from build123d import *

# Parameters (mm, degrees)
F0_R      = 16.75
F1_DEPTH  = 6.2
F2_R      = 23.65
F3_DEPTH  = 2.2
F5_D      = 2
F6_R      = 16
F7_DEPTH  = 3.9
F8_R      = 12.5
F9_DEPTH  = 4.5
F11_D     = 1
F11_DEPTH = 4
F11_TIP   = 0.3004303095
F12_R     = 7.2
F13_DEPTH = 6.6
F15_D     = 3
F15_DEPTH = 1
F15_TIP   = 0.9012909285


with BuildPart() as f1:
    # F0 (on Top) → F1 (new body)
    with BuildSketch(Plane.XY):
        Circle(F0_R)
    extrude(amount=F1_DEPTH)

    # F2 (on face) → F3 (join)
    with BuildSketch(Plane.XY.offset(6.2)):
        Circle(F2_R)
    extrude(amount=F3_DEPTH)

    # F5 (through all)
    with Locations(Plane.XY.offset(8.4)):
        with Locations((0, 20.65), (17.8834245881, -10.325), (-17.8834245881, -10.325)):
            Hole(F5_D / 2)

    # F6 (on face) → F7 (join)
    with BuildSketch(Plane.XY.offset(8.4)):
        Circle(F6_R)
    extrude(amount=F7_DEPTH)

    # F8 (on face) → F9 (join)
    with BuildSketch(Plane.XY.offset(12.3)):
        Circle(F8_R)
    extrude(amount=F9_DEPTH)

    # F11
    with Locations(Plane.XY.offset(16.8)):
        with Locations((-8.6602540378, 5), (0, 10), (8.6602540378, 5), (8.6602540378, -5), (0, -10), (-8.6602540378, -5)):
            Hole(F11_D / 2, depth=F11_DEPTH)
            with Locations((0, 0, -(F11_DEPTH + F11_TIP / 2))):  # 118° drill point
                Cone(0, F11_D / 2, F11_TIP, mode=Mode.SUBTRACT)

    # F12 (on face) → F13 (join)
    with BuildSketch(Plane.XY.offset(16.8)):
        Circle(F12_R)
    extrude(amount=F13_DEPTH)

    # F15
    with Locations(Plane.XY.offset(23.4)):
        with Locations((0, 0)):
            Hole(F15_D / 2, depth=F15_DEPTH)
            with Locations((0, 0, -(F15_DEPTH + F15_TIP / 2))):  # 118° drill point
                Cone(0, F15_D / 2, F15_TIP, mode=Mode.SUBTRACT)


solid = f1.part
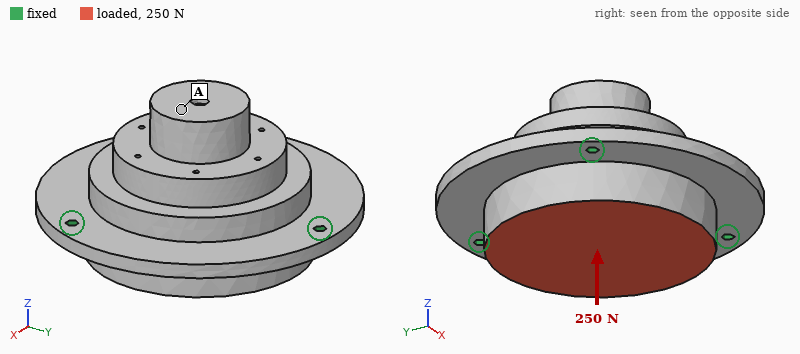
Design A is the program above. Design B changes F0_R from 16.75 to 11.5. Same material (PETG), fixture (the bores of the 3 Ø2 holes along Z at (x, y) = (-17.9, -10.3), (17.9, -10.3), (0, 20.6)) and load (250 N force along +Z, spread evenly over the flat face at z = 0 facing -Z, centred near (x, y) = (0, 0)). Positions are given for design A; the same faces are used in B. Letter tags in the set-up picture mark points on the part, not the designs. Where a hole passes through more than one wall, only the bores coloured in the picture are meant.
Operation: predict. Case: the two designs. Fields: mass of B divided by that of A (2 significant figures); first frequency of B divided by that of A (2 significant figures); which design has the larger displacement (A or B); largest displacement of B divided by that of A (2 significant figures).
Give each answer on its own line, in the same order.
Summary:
0.82
0.90
B
1.6
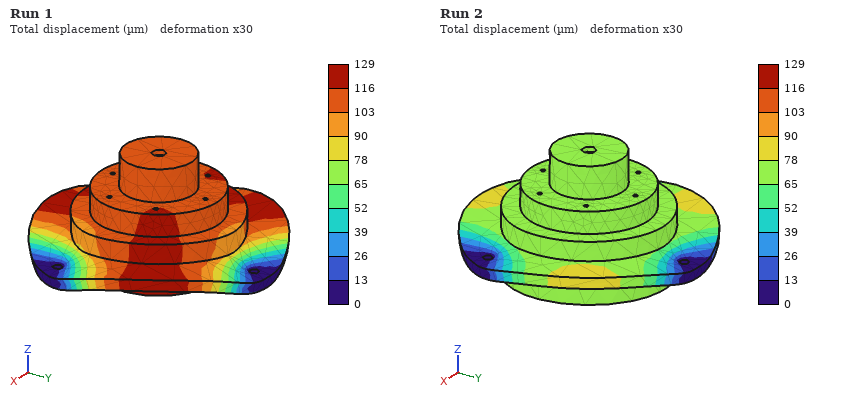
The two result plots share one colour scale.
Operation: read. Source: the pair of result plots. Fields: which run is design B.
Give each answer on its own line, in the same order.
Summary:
Run 1
